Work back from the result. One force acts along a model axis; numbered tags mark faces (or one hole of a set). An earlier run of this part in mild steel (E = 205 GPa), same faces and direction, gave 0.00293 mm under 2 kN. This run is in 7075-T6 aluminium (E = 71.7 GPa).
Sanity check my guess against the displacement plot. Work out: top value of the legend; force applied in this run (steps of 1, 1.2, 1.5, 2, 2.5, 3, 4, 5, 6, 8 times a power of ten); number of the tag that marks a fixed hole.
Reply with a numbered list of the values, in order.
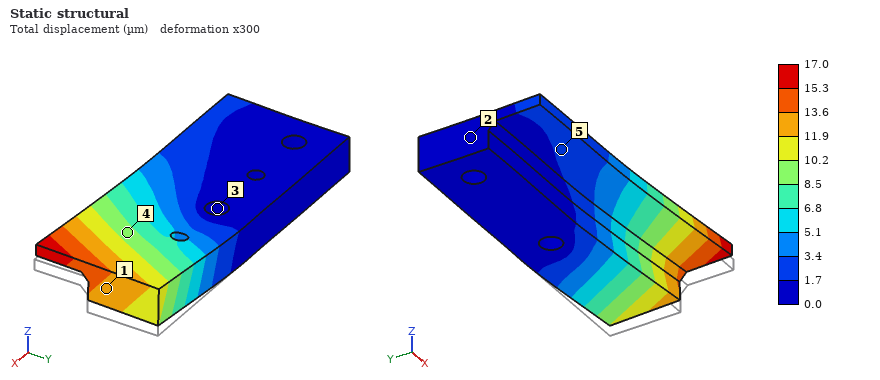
1. 17.0 µm
2. 4 kN
3. 3
